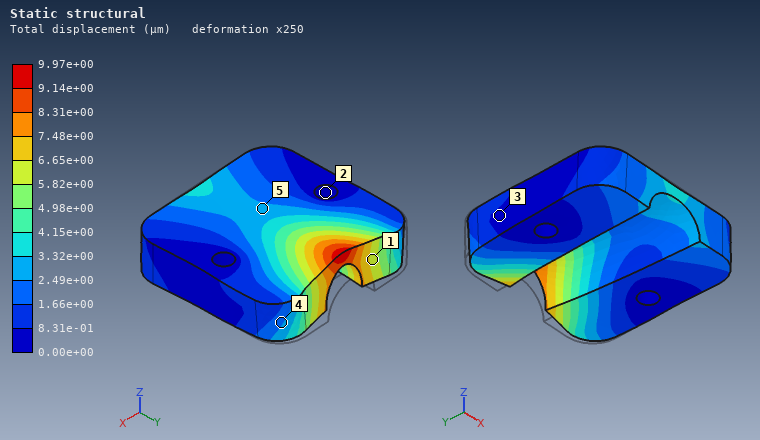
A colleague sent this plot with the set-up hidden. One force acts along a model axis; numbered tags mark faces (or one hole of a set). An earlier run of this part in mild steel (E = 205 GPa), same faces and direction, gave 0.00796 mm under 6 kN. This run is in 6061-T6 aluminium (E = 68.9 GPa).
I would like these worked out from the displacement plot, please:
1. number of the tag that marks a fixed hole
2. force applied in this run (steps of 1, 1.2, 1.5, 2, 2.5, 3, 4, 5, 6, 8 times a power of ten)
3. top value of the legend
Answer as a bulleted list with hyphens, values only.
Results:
- 2
- 2.5 kN
- 9.97e+00 µm
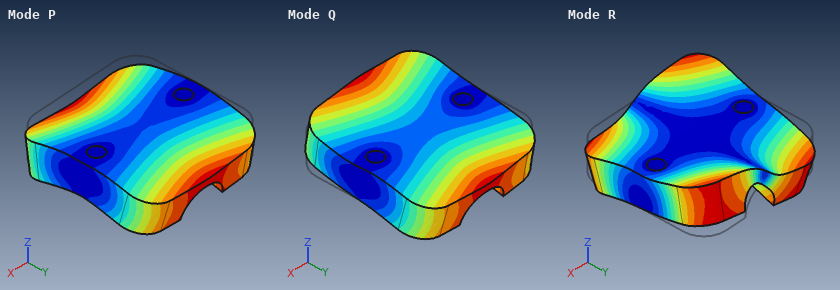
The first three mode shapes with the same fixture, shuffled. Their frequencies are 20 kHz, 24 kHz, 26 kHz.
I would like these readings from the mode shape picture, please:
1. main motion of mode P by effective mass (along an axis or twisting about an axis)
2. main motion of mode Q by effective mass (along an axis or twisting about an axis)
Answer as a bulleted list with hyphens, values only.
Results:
- along Z
- twisting about X
